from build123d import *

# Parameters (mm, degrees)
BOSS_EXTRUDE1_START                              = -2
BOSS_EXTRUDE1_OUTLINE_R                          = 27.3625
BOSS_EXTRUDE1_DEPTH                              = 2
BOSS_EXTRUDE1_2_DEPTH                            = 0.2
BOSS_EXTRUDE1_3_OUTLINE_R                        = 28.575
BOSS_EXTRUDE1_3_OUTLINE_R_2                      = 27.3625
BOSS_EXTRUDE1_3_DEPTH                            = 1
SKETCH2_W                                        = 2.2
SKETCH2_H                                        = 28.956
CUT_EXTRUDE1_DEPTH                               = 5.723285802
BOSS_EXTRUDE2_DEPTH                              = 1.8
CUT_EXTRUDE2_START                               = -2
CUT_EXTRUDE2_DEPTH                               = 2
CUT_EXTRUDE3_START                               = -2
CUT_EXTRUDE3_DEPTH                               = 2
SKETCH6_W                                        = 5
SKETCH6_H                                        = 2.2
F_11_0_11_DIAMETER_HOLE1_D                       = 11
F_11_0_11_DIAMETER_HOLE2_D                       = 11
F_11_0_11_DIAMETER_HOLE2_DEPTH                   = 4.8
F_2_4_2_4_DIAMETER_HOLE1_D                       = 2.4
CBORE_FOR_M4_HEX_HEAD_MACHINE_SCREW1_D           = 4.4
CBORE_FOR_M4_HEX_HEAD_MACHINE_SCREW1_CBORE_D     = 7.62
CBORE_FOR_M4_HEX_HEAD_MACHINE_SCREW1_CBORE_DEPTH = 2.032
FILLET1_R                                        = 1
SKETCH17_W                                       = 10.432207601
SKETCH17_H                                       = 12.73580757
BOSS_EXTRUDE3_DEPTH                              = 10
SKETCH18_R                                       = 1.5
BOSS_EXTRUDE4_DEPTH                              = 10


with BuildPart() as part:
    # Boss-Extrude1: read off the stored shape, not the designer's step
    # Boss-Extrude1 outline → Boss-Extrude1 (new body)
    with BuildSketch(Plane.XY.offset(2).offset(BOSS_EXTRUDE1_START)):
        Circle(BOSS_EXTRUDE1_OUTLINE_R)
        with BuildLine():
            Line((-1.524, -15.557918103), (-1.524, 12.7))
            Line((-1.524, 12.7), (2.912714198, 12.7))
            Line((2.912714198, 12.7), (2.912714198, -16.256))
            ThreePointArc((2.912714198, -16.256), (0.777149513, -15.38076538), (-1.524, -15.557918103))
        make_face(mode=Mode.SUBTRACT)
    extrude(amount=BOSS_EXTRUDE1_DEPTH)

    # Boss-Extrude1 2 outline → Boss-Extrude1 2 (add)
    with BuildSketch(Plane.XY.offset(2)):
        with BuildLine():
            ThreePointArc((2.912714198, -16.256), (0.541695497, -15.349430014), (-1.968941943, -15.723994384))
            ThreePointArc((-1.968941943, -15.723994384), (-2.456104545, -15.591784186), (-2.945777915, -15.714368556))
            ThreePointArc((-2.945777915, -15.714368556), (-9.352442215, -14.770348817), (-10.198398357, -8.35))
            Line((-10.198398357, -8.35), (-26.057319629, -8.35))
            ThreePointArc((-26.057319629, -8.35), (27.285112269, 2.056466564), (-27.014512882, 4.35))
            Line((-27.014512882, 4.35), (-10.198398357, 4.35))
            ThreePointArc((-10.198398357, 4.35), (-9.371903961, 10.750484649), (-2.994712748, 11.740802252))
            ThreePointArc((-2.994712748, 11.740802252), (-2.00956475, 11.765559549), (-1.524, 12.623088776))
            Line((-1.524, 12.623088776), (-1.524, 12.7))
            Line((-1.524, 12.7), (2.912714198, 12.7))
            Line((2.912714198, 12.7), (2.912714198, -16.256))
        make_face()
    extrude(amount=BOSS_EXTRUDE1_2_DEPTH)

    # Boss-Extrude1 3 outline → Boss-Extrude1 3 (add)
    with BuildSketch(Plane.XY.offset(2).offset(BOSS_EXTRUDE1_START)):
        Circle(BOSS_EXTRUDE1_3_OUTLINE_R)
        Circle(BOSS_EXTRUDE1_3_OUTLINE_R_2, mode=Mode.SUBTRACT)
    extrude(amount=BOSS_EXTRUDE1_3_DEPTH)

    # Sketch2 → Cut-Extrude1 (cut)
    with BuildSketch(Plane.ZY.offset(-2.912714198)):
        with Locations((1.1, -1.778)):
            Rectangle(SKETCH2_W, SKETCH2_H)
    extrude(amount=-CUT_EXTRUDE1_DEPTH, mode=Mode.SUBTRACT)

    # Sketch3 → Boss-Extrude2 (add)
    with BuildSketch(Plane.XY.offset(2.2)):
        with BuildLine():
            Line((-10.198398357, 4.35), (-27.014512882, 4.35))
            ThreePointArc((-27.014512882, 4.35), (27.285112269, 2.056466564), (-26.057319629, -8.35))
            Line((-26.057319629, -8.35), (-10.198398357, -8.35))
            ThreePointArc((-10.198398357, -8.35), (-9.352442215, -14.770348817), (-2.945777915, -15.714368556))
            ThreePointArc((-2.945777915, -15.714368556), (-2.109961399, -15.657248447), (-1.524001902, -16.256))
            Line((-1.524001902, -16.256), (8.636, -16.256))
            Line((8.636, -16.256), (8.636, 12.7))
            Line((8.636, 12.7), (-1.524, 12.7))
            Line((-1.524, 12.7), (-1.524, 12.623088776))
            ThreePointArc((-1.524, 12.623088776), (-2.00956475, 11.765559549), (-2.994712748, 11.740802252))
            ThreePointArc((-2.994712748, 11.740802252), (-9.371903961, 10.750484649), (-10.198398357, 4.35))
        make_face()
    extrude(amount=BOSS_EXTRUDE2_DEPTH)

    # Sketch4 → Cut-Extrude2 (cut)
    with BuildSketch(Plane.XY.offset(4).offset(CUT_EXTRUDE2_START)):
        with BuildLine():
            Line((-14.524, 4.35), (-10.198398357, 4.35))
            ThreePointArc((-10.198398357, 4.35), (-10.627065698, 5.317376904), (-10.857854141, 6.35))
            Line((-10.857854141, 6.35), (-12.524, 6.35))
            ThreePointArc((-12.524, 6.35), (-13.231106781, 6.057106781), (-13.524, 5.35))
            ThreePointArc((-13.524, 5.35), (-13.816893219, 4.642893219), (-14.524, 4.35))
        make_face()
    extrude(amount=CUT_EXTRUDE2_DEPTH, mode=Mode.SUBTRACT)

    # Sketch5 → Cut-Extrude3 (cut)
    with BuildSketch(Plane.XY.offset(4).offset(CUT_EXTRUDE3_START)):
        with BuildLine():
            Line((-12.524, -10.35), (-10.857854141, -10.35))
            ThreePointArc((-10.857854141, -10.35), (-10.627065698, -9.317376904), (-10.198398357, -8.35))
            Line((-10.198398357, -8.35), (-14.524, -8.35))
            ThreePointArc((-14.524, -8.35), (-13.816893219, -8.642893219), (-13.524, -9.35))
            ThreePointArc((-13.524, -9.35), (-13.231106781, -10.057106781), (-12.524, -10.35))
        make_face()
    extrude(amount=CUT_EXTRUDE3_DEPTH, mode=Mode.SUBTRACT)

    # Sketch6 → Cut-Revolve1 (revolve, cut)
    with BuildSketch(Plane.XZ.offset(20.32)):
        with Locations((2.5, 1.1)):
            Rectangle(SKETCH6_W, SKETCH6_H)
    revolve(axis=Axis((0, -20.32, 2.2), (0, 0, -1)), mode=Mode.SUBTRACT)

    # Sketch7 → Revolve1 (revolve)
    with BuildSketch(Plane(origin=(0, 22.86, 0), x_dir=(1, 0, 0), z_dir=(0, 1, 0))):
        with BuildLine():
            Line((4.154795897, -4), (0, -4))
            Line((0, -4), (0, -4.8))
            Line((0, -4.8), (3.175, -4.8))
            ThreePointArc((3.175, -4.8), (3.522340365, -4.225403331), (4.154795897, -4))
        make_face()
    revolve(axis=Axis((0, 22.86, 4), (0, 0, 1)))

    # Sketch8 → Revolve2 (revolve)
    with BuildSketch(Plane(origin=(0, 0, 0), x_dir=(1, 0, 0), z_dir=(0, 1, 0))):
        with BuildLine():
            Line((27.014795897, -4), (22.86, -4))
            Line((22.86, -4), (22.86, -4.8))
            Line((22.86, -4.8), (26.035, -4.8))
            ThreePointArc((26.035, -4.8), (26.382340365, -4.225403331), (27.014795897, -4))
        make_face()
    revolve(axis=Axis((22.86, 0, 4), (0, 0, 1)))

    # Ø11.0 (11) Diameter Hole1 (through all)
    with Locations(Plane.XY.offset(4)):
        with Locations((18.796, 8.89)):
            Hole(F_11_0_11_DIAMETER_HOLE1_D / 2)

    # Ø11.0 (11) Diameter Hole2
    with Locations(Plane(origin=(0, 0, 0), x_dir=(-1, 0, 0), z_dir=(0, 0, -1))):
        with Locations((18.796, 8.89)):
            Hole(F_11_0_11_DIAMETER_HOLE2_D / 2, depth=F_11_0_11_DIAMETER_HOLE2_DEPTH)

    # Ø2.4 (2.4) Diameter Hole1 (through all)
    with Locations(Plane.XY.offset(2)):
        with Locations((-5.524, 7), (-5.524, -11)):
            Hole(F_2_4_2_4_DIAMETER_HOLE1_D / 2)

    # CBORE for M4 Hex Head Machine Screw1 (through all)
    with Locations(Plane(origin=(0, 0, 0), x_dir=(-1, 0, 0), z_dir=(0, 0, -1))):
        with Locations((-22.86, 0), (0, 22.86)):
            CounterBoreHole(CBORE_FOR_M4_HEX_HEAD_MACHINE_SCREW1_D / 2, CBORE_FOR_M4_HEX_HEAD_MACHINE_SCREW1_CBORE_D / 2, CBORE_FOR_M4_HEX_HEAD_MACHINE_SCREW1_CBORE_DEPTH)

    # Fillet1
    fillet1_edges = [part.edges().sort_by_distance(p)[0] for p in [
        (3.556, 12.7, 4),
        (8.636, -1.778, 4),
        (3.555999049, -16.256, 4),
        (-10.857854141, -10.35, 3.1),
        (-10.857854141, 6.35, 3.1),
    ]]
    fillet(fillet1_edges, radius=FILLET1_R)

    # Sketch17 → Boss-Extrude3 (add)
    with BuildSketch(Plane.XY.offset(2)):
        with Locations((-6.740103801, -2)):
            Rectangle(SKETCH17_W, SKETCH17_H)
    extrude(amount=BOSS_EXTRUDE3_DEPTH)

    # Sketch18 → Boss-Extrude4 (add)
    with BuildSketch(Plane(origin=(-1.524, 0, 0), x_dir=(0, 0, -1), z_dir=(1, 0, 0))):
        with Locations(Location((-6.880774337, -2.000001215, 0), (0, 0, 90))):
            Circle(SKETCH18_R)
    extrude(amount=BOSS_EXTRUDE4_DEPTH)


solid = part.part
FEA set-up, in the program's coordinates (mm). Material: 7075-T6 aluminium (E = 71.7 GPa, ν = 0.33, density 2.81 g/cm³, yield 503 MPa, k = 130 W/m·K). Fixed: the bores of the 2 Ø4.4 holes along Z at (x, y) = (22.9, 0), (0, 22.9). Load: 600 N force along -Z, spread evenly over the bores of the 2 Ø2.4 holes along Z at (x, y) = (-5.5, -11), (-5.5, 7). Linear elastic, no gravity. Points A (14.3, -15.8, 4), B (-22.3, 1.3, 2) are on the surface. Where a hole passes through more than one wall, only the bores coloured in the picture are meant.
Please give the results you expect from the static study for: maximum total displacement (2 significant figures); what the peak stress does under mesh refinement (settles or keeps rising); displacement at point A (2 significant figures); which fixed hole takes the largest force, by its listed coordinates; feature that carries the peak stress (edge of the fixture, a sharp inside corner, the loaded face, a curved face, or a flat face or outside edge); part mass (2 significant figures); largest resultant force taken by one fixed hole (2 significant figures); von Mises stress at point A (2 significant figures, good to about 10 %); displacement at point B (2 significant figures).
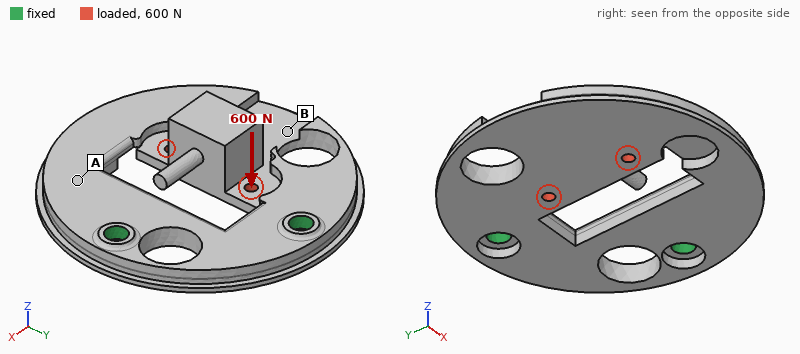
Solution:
0.68 mm
keeps rising
0.16 mm
(0, 22.9)
a sharp inside corner
22 g
400 N
79 MPa
0.41 mm
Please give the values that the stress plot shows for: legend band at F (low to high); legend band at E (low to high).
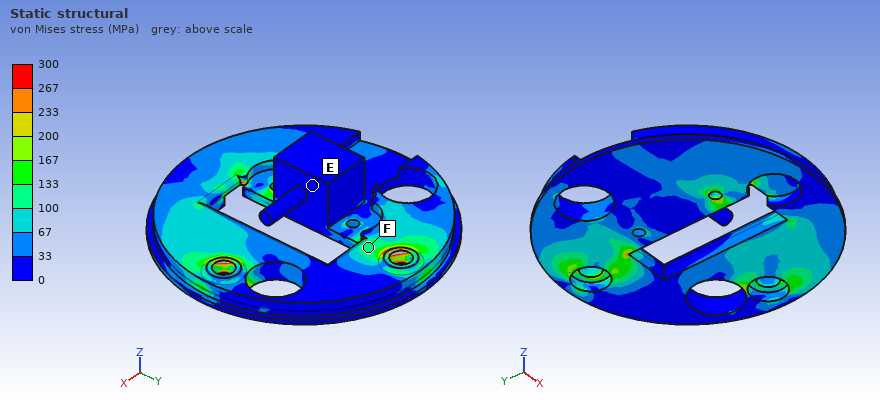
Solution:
100 to 133 MPa
0 to 33 MPa
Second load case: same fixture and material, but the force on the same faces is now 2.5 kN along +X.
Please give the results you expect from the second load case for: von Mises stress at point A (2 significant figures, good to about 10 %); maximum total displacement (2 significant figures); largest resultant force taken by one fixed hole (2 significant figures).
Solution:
40 MPa
0.30 mm
1.6 kN
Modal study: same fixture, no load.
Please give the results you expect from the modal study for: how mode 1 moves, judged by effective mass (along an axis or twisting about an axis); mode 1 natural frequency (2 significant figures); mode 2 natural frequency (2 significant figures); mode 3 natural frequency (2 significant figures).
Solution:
along Z
1400 Hz
3400 Hz
4900 Hz
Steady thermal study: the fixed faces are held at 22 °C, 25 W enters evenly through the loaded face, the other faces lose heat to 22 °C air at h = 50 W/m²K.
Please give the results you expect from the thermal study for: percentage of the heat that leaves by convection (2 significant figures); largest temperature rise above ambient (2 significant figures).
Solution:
30 %
62 K
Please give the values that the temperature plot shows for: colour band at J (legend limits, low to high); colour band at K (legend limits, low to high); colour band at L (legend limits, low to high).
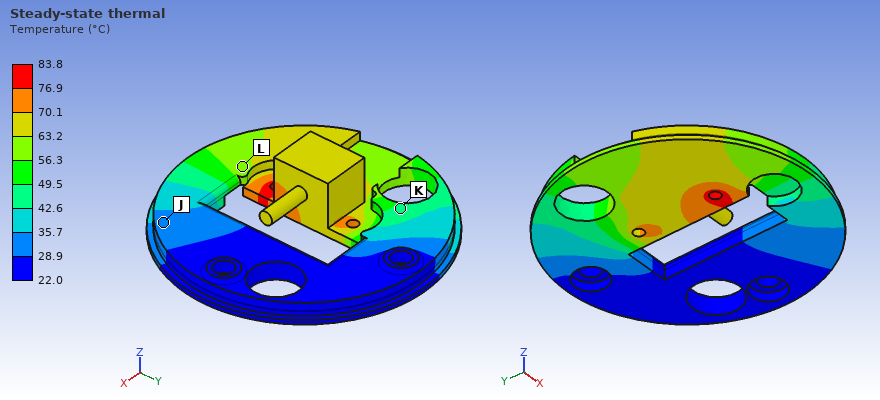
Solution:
28.9 to 35.7 °C
42.6 to 49.5 °C
56.3 to 63.2 °C
